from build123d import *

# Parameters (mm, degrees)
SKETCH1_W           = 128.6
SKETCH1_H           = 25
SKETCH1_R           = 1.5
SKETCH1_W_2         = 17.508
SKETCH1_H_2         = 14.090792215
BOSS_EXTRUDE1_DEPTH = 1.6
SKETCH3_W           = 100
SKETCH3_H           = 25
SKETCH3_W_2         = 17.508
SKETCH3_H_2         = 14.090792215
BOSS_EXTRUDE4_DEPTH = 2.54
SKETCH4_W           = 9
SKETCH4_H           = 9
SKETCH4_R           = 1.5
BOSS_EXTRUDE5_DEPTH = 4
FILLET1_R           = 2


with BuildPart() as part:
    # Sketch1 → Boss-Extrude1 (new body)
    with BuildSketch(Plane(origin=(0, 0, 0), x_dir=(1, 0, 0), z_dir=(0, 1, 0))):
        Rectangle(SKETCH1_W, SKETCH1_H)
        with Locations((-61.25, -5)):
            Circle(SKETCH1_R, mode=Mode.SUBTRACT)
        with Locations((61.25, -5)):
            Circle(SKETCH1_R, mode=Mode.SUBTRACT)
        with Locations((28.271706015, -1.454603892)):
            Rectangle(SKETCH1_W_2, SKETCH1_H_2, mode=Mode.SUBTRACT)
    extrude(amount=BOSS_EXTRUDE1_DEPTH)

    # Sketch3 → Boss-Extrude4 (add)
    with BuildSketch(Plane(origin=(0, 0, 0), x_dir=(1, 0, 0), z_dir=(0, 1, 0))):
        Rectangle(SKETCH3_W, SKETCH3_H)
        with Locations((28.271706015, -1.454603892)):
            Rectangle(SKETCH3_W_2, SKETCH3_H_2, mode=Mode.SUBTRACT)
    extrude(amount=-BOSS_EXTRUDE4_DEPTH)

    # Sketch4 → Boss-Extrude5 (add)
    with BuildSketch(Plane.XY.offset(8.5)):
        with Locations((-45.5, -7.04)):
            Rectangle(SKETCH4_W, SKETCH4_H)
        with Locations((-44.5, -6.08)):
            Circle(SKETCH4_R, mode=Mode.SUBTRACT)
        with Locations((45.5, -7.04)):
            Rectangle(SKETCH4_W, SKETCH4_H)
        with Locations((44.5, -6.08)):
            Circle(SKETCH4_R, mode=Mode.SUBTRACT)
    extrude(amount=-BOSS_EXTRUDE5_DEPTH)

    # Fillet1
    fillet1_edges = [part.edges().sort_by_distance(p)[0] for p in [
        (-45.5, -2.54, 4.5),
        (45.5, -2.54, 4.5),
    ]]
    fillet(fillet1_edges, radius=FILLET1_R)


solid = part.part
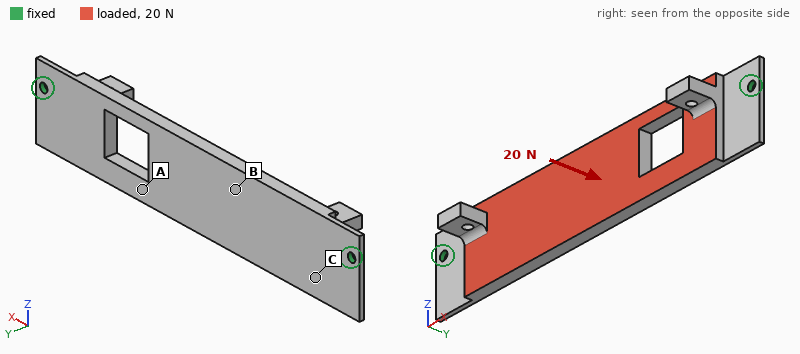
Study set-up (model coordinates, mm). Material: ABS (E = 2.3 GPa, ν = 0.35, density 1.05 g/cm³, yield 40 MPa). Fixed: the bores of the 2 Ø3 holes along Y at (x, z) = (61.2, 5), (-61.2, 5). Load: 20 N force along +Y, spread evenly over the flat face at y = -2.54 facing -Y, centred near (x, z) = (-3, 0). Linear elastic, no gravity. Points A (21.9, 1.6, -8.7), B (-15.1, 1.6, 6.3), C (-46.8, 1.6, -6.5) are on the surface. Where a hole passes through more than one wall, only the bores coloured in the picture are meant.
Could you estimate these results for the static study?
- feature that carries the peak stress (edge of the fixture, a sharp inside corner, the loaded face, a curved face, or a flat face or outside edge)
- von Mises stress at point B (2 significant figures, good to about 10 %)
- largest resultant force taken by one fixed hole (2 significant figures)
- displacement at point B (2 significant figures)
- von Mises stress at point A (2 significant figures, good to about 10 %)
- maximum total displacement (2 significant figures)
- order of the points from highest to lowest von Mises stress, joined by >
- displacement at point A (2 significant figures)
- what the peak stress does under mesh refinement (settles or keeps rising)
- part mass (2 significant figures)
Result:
edge of the fixture
2.3 MPa
48 N
0.90 mm
4.2 MPa
1.4 mm
A > B > C
1.2 mm
keeps rising
12 g
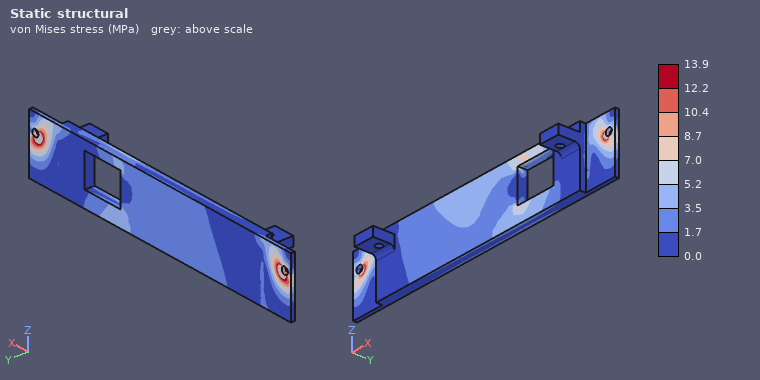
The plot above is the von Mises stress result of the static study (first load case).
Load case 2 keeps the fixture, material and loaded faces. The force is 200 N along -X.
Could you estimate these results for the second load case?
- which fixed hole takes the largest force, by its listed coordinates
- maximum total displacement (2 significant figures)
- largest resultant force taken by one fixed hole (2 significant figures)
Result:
(-61.2, 5)
0.14 mm
110 N
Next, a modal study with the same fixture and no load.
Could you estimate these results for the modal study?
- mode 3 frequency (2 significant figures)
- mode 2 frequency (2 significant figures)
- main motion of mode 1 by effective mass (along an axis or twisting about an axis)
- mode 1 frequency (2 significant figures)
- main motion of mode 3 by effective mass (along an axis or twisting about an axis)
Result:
690 Hz
430 Hz
along Y
230 Hz
twisting about Z
